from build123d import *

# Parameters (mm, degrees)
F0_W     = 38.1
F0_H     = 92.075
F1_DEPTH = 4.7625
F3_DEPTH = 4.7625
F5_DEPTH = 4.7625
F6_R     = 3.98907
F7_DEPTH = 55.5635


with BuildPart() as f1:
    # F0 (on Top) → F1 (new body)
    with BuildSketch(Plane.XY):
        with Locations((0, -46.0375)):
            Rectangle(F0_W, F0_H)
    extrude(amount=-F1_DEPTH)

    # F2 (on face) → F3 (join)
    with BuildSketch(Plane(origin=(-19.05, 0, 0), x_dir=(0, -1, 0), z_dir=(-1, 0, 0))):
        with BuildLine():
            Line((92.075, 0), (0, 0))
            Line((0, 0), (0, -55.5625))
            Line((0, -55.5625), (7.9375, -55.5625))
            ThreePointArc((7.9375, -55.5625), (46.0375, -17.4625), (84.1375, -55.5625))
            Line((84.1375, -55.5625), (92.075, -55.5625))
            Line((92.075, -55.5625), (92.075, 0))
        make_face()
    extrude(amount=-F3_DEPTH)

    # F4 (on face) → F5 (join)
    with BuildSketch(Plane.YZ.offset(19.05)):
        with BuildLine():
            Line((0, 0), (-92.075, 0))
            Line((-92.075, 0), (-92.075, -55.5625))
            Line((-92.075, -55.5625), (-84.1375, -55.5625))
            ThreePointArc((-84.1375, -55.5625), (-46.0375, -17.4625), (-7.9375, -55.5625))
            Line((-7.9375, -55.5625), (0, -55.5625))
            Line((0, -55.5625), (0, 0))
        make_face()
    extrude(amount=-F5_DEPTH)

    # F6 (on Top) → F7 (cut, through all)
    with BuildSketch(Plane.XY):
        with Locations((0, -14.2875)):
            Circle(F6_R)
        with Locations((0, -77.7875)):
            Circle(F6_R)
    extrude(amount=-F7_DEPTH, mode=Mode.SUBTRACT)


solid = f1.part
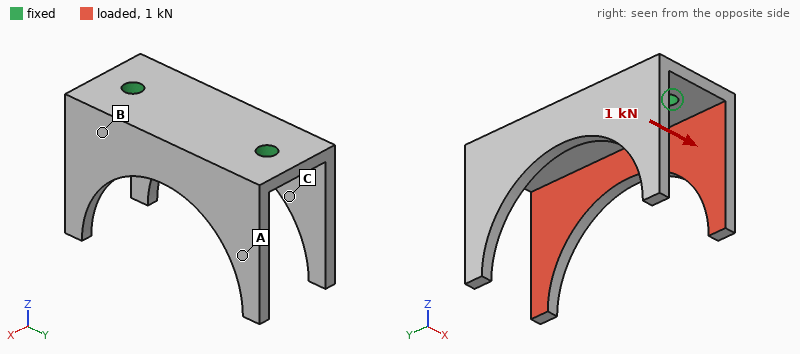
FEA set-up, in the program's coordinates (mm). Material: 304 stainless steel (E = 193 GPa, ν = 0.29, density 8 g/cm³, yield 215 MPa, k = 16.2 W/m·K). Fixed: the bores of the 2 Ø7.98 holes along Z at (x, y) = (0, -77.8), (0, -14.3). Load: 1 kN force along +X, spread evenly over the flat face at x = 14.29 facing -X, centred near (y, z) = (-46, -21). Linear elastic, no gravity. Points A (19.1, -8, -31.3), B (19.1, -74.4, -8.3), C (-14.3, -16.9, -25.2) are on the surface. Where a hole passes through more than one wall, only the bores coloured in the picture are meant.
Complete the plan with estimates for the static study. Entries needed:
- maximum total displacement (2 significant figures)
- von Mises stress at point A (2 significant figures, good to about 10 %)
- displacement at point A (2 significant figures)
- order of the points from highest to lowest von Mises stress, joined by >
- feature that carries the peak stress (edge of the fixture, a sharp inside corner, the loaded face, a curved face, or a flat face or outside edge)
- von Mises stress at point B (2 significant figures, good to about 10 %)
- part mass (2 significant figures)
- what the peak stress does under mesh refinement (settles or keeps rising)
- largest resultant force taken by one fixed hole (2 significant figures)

0.21 mm
23 MPa
0.097 mm
B > A > C
edge of the fixture
41 MPa
310 g
keeps rising
500 N
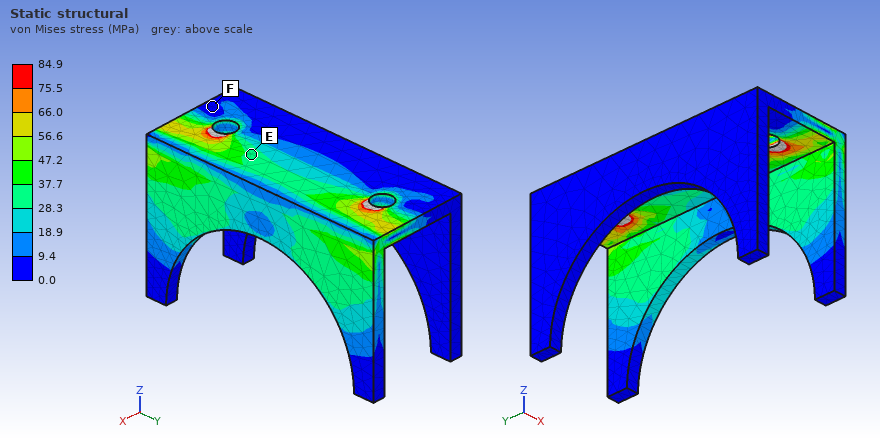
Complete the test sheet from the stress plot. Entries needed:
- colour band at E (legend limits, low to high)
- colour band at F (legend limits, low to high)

28.3 to 37.7 MPa
0.0 to 9.4 MPa
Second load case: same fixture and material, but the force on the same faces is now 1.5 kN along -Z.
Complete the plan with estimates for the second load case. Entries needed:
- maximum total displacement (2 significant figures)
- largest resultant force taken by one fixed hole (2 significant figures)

32 µm
750 N
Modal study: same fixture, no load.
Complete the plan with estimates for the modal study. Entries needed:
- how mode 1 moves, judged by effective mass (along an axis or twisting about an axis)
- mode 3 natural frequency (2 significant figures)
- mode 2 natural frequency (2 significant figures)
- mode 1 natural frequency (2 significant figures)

along X
1700 Hz
1600 Hz
1500 Hz
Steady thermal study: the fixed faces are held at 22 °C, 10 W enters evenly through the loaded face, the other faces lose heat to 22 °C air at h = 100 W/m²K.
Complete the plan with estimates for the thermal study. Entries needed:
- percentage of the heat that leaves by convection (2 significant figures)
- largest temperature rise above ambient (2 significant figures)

78 %
19 K
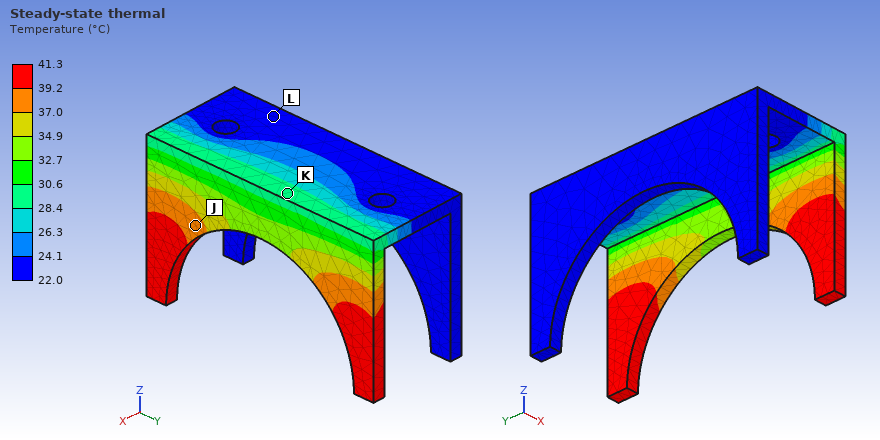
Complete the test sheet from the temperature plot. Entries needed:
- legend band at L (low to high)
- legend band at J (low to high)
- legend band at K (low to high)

22.0 to 24.1 °C
37.0 to 39.2 °C
28.4 to 30.6 °C
